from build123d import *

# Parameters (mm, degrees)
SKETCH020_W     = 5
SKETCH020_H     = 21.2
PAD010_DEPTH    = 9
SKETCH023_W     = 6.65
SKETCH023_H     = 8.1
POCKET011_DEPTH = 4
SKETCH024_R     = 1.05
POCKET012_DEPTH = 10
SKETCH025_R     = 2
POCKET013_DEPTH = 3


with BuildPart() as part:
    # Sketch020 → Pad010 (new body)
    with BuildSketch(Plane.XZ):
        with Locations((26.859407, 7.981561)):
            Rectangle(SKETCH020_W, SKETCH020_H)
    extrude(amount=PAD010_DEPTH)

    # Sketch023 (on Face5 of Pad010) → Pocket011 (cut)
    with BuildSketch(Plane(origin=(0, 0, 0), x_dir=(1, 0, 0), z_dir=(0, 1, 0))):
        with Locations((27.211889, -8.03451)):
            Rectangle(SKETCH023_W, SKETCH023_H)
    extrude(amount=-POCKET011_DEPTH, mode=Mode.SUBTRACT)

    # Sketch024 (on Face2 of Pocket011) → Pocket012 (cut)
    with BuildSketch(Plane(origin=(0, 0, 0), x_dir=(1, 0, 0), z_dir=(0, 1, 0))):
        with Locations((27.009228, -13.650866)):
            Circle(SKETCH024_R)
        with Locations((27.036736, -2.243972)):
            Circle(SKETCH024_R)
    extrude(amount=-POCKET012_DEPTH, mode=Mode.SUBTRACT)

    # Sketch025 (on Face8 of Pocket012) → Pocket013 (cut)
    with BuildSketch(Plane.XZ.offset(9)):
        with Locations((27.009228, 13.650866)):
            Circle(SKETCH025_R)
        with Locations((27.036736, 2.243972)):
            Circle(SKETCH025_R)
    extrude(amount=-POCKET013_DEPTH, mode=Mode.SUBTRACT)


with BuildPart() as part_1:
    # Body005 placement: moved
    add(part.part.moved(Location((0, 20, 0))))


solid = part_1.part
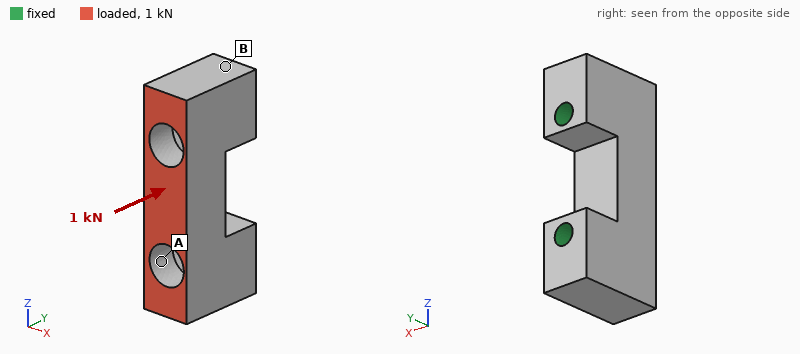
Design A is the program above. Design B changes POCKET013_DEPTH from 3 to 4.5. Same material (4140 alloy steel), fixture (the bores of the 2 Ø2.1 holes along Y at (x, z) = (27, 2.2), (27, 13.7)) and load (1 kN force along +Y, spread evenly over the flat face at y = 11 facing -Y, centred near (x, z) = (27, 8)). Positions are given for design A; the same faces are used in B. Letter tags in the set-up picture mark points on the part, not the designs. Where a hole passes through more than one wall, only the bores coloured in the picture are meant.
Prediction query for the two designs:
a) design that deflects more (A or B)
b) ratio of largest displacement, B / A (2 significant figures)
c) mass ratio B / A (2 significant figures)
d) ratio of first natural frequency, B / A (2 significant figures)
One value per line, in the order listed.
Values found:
B
1.5
0.96
0.66
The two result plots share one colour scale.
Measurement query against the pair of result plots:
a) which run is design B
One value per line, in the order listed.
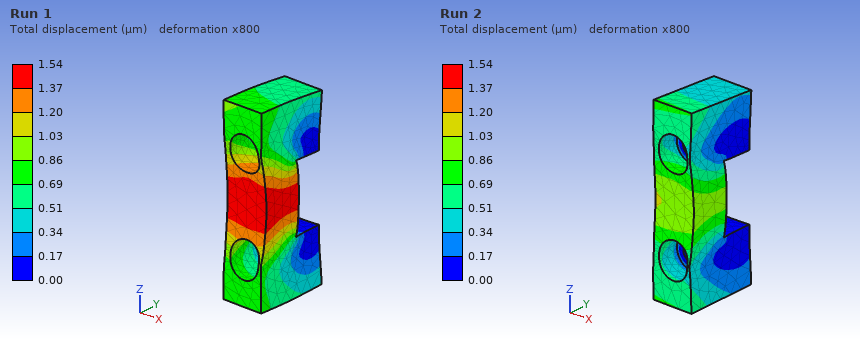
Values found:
Run 1
